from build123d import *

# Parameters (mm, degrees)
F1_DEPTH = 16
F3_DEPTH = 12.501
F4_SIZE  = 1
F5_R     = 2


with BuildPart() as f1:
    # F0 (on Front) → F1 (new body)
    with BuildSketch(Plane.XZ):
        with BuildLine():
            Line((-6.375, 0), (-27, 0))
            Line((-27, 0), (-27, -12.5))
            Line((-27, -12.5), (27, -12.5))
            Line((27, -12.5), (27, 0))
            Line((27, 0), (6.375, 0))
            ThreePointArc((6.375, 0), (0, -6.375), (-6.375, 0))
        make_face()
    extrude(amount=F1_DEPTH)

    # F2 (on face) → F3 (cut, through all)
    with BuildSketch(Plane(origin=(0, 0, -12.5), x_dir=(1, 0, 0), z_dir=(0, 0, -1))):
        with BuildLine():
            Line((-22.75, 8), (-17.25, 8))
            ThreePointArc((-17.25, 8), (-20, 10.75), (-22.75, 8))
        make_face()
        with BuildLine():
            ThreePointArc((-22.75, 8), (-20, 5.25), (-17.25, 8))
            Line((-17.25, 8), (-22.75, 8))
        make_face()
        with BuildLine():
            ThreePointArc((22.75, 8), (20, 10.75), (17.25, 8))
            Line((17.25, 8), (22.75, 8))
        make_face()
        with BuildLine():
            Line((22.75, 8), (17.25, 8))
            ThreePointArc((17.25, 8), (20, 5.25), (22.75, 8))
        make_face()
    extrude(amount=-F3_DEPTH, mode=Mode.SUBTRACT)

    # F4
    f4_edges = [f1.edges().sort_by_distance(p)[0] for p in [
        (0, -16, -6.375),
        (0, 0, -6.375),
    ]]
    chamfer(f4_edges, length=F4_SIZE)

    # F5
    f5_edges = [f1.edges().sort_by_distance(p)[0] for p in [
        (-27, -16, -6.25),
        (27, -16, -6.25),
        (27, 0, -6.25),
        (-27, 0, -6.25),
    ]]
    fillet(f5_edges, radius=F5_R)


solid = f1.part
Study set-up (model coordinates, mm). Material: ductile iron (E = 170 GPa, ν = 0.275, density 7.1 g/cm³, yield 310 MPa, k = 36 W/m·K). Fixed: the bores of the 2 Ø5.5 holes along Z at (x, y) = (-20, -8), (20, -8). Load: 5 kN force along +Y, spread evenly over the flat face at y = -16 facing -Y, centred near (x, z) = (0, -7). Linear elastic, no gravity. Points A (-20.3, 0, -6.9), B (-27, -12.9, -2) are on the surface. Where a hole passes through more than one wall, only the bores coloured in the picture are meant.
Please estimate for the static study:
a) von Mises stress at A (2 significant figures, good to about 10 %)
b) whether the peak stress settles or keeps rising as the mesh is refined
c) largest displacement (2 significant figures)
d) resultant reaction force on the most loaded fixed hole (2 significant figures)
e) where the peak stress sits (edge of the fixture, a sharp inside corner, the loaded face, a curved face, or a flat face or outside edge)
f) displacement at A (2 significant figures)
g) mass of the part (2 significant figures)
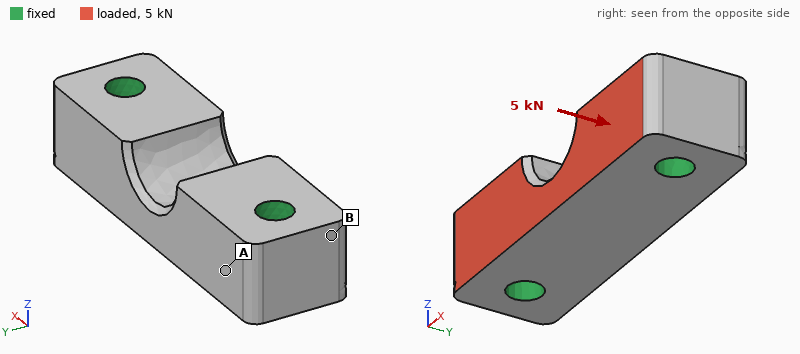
9.2 MPa
keeps rising
3.8 µm
2.5 kN
edge of the fixture
0.70 µm
65 g
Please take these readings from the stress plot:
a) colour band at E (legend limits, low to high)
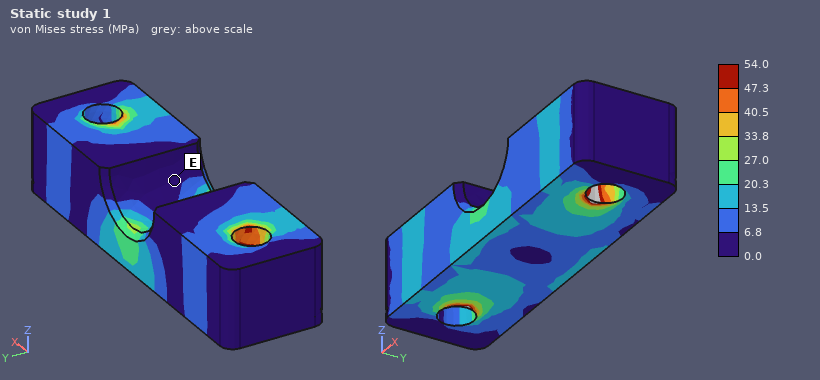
0.0 to 6.8 MPa
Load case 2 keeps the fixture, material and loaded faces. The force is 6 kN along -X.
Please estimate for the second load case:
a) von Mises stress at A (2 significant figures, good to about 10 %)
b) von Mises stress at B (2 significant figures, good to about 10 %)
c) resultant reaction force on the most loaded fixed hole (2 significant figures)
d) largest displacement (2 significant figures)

5.0 MPa
11 MPa
3.1 kN
2.2 µm
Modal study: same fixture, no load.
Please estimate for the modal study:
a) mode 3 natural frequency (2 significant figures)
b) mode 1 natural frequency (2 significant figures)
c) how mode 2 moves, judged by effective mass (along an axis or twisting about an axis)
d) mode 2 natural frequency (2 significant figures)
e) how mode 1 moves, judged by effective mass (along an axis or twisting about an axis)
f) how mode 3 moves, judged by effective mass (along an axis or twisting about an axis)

42 kHz
27 kHz
along Z
29 kHz
along Y
twisting about X
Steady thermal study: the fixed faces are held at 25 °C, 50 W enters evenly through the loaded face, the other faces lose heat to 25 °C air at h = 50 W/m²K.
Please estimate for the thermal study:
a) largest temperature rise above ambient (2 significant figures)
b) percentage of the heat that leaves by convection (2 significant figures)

36 K
3.1 %
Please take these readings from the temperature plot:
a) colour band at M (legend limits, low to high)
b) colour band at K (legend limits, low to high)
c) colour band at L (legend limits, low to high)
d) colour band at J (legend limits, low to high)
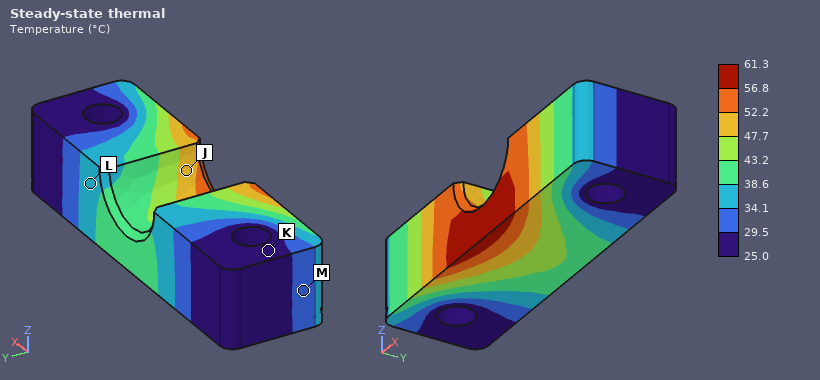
29.5 to 34.1 °C
25.0 to 29.5 °C
34.1 to 38.6 °C
47.7 to 52.2 °C
